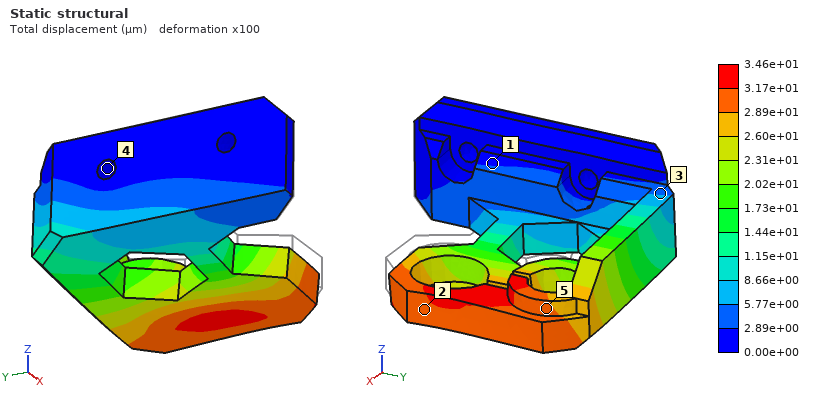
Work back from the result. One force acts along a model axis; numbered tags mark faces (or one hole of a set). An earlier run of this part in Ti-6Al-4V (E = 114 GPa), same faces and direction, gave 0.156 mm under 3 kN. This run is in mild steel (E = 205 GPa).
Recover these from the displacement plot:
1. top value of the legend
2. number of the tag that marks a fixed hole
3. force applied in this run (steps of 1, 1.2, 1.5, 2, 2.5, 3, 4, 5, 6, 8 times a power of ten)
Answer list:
3.46e+01 µm
4
1.2 kN
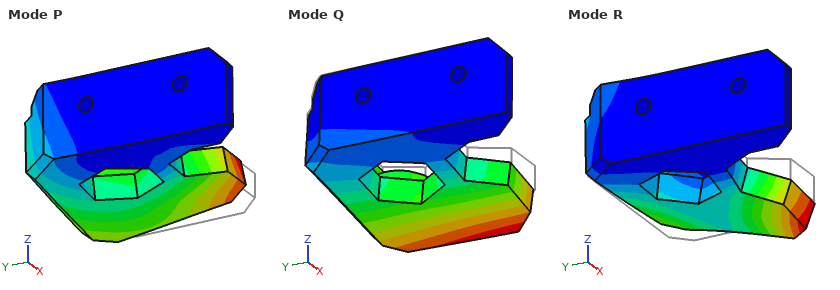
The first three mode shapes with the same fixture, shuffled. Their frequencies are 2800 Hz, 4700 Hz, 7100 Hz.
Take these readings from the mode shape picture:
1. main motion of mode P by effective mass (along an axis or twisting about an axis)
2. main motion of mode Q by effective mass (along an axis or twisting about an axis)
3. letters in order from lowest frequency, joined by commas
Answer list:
along Y
along Z
Q, P, R
